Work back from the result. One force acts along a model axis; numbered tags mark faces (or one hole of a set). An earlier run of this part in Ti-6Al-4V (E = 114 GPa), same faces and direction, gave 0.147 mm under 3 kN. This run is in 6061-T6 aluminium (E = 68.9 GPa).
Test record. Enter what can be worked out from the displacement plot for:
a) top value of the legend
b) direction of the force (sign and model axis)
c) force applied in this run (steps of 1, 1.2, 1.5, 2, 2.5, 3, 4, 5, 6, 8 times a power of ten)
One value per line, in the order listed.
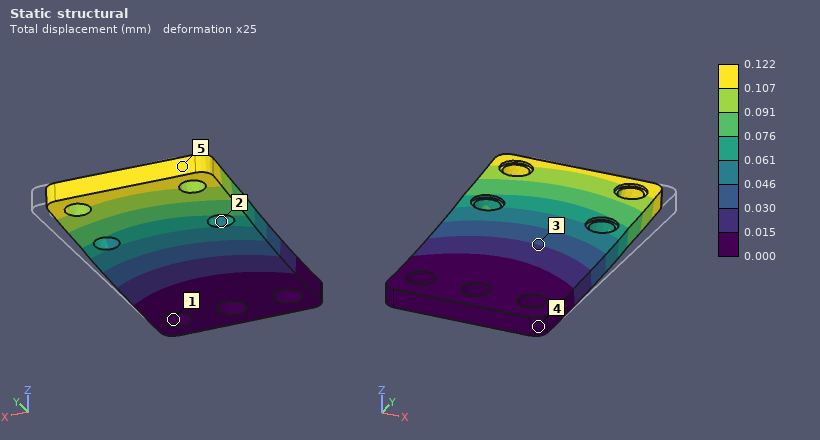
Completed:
0.122 mm
-X
1.5 kN
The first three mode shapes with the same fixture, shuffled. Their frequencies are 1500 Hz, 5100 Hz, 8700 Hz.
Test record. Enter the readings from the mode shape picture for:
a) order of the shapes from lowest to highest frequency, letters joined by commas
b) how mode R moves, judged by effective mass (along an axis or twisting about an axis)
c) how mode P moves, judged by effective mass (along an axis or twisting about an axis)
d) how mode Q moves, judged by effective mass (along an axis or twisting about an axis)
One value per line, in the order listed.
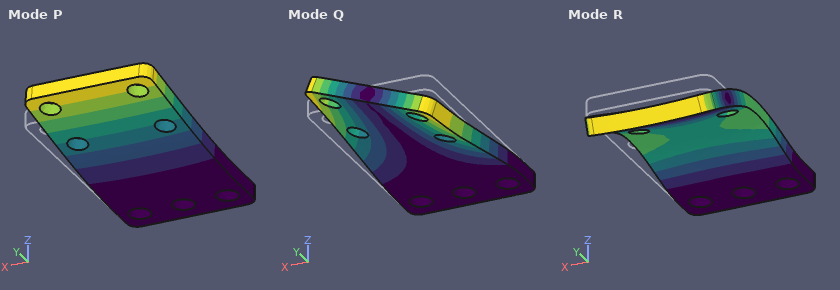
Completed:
P, Q, R
along Z
along Z
twisting about Y
